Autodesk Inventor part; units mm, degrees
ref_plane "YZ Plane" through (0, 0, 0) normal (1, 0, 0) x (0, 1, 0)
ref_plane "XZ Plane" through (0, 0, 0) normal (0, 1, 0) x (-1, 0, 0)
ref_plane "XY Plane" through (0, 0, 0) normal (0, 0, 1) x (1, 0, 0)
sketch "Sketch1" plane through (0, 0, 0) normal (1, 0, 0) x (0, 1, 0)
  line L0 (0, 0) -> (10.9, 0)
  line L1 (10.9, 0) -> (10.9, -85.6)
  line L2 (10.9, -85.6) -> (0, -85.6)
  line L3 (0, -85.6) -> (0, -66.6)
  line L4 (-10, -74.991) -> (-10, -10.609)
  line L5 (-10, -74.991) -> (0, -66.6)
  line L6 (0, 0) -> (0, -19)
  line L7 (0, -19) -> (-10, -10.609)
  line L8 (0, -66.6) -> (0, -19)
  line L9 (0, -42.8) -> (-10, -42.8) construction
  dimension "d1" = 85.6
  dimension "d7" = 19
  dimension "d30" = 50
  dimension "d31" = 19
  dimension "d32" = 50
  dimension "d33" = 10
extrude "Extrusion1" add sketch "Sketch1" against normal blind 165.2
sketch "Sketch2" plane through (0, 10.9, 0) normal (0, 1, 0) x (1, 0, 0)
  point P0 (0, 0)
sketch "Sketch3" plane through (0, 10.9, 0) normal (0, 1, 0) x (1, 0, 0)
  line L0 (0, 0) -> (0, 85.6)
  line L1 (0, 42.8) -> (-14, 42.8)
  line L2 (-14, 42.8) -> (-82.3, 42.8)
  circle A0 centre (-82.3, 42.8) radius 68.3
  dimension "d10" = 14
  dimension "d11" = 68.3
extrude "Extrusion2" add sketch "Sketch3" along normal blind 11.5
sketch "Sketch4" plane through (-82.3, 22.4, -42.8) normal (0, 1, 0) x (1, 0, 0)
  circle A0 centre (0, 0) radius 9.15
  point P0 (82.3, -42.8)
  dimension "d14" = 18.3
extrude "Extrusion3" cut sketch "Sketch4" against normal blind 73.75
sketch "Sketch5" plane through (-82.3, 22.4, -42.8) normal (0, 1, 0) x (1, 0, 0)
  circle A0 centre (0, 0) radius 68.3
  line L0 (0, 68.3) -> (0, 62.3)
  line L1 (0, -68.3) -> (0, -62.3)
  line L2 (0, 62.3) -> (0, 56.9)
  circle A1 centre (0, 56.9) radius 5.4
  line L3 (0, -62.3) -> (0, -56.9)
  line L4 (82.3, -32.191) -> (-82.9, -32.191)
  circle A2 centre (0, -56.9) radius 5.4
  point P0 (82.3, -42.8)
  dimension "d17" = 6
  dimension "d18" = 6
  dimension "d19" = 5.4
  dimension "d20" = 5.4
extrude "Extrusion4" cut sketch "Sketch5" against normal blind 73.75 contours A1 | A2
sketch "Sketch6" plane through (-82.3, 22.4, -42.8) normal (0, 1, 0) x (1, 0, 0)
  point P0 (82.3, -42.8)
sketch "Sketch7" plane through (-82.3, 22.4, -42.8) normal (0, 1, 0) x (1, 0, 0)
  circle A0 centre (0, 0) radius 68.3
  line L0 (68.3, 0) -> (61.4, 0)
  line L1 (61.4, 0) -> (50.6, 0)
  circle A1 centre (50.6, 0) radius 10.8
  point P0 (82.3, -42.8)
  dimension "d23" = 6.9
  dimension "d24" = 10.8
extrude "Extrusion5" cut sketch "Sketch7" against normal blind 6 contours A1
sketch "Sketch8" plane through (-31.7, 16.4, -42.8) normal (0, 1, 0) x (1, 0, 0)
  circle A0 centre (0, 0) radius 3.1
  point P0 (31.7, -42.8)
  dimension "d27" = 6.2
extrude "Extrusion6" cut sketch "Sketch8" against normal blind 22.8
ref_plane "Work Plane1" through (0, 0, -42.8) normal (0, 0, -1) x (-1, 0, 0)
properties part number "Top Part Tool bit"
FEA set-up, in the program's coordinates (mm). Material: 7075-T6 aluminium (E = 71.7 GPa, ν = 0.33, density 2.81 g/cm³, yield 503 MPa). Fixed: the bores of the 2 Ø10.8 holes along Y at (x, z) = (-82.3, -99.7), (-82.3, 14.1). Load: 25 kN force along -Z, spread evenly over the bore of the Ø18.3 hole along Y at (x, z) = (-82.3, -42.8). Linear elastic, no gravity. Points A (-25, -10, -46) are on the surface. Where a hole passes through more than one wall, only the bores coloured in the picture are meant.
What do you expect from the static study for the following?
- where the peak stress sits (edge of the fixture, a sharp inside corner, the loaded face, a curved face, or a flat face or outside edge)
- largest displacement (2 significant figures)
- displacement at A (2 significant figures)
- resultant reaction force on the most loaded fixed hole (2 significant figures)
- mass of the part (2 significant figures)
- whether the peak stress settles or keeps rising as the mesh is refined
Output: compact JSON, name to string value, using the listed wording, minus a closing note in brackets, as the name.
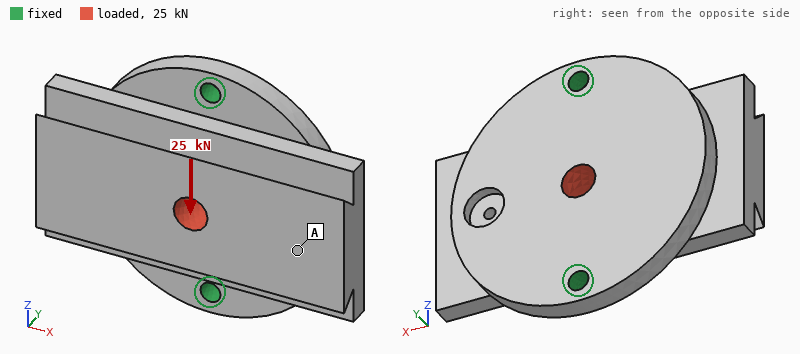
{"where the peak stress sits": "edge of the fixture", "largest displacement": "20 µm", "displacement at A": "12 µm", "resultant reaction force on the most loaded fixed hole": "13 kN", "mass of the part": "1.1 kg", "whether the peak stress settles or keeps rising as the mesh is refined": "keeps rising"}
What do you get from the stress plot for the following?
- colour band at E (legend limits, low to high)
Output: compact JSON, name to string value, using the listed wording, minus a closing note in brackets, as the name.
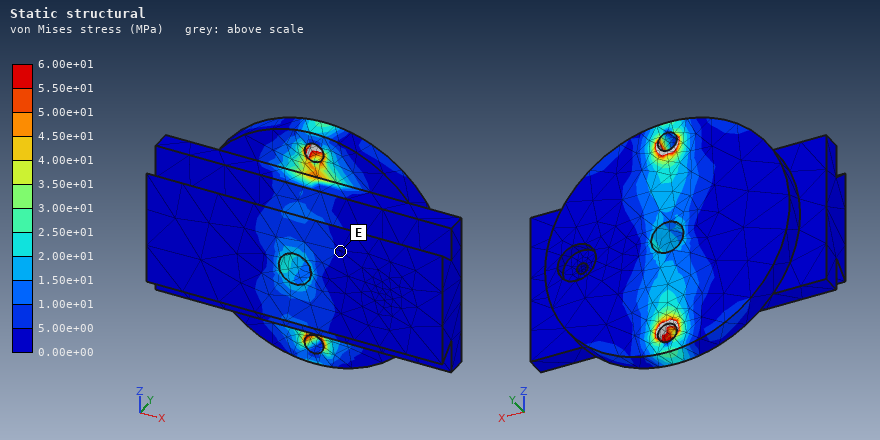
{"colour band at E": "0.00e+00 to 5.00e+00 MPa"}
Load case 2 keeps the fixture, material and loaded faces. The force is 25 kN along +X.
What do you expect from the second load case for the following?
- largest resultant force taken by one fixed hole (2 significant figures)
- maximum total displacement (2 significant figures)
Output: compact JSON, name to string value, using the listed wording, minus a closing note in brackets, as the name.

{"largest resultant force taken by one fixed hole": "13 kN", "maximum total displacement": "0.27 mm"}
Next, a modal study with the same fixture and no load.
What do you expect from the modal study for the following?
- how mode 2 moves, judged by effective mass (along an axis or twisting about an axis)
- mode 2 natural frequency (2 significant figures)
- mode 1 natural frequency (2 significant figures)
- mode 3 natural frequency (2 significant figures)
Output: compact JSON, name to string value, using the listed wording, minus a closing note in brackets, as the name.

{"how mode 2 moves, judged by effective mass": "along Y", "mode 2 natural frequency": "2600 Hz", "mode 1 natural frequency": "1000 Hz", "mode 3 natural frequency": "5500 Hz"}
